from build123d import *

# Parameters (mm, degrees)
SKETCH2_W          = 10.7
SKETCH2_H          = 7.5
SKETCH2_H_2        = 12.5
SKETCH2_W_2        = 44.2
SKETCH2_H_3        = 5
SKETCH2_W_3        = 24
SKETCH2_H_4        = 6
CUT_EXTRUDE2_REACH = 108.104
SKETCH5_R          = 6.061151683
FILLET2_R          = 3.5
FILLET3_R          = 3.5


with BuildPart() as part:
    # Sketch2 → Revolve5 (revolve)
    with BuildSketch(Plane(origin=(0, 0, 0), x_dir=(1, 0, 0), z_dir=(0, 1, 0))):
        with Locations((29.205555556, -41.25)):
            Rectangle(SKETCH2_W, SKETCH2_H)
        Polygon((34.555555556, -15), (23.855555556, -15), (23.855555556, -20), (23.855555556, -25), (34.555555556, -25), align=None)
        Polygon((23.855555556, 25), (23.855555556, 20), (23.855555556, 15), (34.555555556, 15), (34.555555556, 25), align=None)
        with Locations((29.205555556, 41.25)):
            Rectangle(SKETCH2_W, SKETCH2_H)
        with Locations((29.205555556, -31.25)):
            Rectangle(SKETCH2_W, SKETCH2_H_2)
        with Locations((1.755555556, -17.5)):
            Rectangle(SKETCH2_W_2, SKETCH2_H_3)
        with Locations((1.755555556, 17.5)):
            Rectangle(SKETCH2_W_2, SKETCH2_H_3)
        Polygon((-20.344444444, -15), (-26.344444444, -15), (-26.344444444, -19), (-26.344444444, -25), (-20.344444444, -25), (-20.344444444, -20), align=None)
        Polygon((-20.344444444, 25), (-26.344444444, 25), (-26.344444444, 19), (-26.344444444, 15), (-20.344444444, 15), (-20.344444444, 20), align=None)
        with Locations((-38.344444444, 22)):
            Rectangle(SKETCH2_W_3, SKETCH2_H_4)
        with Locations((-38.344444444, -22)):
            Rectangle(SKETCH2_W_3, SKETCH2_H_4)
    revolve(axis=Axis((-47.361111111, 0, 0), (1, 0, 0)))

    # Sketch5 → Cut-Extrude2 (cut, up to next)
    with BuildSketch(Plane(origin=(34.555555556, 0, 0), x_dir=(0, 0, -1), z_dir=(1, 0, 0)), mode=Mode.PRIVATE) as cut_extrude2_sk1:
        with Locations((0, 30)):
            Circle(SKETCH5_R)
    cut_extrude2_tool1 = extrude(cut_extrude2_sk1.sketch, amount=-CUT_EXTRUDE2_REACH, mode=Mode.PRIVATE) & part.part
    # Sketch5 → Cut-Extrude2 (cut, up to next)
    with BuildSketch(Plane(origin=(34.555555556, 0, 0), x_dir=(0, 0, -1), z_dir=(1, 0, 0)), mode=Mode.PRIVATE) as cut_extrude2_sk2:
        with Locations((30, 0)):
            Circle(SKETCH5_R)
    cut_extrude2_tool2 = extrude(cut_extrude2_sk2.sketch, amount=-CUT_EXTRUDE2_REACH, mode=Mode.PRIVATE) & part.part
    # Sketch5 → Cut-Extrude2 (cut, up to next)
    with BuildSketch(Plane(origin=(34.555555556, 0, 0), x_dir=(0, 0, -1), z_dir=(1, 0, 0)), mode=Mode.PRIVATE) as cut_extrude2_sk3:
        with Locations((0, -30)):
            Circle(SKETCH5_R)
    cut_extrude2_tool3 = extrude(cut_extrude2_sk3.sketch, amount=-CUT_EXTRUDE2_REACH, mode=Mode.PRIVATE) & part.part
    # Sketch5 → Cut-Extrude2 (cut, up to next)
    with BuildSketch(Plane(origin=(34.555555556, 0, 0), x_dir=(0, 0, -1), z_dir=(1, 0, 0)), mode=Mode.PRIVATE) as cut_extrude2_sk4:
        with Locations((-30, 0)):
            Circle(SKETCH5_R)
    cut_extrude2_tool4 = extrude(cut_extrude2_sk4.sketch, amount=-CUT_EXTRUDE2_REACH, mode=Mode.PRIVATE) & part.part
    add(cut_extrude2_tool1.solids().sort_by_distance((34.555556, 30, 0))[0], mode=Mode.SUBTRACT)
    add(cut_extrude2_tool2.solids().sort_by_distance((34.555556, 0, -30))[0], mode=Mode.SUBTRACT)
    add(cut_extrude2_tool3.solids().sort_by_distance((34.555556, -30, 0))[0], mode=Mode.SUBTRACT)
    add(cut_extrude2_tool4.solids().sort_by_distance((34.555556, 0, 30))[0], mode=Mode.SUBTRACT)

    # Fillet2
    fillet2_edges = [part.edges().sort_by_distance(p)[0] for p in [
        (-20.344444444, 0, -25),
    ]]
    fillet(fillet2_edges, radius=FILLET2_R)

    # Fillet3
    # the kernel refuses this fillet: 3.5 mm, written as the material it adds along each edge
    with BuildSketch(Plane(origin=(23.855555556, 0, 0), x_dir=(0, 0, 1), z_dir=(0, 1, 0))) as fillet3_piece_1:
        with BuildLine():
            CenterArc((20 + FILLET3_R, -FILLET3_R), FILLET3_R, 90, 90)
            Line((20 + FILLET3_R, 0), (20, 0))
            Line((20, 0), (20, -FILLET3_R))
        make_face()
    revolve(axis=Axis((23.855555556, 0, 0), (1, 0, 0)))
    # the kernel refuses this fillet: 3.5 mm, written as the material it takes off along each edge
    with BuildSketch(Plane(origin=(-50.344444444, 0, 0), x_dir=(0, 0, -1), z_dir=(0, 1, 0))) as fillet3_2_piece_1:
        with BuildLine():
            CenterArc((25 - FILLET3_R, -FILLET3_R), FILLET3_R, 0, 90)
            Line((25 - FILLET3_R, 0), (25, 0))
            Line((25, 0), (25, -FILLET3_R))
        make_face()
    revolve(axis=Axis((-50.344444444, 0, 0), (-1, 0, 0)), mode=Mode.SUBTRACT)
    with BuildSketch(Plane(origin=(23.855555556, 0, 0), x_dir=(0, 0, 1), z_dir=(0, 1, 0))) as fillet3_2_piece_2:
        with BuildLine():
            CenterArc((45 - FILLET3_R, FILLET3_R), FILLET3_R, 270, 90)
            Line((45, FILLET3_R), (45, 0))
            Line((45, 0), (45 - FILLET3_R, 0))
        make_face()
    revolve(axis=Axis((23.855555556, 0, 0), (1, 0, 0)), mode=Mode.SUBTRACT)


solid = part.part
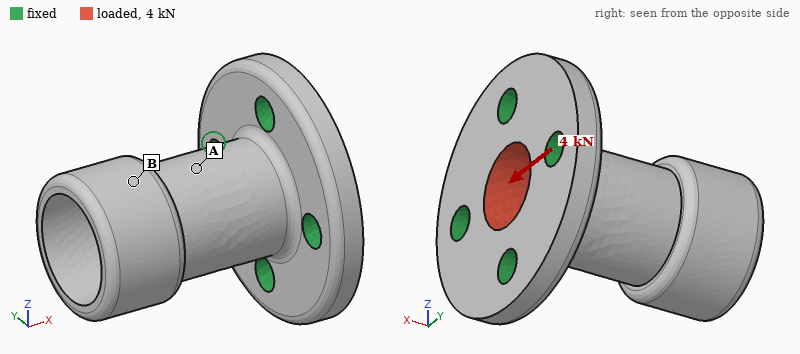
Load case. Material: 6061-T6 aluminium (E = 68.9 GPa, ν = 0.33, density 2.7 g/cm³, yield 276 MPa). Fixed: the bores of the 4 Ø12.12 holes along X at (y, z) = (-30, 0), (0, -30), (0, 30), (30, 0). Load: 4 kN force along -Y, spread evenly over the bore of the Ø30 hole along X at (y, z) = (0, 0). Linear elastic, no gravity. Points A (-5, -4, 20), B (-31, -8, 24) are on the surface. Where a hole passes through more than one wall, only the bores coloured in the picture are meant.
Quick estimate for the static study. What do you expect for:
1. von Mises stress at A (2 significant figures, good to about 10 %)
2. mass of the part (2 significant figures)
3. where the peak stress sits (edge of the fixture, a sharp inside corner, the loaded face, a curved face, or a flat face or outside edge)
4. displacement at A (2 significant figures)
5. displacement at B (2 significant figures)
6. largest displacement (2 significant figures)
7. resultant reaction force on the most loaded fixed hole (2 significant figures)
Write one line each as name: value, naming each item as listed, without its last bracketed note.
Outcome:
von Mises stress at A: 8.0 MPa
mass of the part: 290 g
where the peak stress sits: a curved face
displacement at A: 17 µm
displacement at B: 29 µm
largest displacement: 37 µm
resultant reaction force on the most loaded fixed hole: 2.3 kN
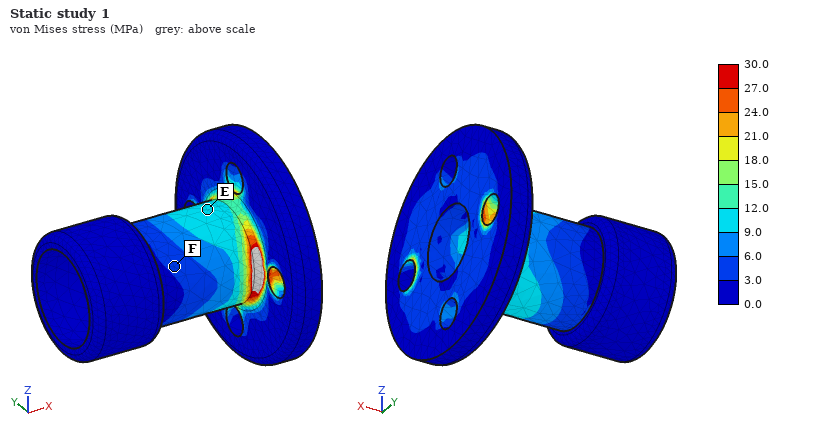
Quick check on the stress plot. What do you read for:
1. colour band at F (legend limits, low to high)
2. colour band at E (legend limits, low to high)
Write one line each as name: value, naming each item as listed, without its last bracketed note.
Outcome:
colour band at F: 3.0 to 6.0 MPa
colour band at E: 9.0 to 12.0 MPa
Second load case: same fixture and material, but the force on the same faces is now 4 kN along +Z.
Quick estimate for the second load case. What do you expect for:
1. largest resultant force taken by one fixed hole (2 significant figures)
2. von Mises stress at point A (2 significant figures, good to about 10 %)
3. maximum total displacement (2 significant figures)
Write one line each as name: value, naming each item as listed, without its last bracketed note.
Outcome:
largest resultant force taken by one fixed hole: 2.3 kN
von Mises stress at point A: 4.2 MPa
maximum total displacement: 37 µm
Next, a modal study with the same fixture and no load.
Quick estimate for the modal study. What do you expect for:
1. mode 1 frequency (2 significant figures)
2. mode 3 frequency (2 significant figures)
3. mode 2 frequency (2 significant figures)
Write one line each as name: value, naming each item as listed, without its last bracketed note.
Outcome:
mode 1 frequency: 3400 Hz
mode 3 frequency: 7300 Hz
mode 2 frequency: 3400 Hz
